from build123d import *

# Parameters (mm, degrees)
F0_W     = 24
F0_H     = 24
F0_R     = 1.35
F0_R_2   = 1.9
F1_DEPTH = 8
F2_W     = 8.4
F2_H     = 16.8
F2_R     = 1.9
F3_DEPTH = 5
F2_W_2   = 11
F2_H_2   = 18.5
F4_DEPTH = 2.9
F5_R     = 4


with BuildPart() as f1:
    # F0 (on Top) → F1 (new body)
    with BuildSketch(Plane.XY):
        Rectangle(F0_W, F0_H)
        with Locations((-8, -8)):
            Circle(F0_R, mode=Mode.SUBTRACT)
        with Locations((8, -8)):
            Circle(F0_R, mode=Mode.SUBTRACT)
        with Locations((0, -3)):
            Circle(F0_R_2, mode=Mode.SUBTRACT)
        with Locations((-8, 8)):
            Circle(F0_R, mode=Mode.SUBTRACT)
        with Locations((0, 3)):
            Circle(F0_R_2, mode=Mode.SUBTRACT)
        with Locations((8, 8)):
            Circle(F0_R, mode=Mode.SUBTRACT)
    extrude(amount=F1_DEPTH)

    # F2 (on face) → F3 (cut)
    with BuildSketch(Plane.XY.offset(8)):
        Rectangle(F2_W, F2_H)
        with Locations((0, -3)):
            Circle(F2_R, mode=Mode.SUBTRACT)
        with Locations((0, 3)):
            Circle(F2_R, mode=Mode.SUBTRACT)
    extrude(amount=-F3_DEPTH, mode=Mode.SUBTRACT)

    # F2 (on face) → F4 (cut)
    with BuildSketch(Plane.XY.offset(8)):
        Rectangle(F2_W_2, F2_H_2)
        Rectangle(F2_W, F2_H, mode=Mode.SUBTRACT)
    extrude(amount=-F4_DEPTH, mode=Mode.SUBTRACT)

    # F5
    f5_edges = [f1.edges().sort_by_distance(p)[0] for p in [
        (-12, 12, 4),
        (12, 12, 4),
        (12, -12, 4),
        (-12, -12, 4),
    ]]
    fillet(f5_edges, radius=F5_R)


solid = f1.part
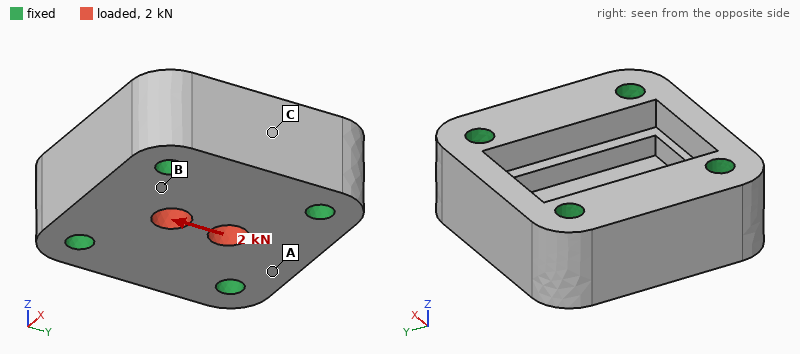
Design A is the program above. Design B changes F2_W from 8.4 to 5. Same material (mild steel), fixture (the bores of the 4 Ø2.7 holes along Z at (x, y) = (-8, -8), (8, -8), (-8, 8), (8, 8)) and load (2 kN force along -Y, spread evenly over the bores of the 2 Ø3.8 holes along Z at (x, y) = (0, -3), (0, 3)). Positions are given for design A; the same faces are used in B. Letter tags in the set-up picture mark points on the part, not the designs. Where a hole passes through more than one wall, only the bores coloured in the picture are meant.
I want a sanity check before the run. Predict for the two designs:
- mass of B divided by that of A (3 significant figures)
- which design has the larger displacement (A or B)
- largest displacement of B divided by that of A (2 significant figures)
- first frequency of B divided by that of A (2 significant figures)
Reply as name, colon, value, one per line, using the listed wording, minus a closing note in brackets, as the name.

mass of B divided by that of A: 1.04
which design has the larger displacement: A
largest displacement of B divided by that of A: 0.90
first frequency of B divided by that of A: 0.99
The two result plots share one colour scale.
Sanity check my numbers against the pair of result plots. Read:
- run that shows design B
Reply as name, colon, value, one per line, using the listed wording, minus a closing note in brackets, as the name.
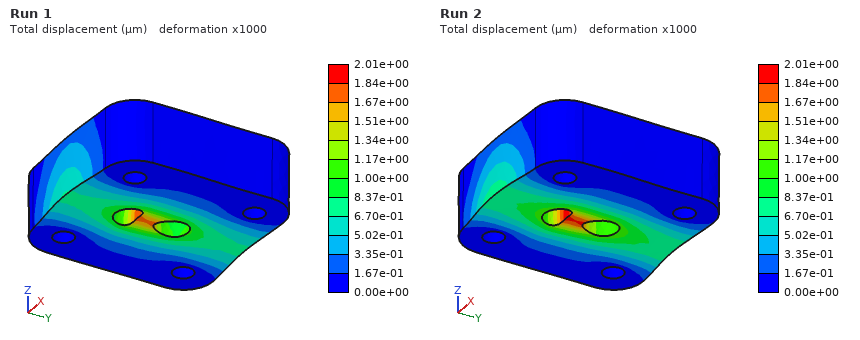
run that shows design B: Run 1
